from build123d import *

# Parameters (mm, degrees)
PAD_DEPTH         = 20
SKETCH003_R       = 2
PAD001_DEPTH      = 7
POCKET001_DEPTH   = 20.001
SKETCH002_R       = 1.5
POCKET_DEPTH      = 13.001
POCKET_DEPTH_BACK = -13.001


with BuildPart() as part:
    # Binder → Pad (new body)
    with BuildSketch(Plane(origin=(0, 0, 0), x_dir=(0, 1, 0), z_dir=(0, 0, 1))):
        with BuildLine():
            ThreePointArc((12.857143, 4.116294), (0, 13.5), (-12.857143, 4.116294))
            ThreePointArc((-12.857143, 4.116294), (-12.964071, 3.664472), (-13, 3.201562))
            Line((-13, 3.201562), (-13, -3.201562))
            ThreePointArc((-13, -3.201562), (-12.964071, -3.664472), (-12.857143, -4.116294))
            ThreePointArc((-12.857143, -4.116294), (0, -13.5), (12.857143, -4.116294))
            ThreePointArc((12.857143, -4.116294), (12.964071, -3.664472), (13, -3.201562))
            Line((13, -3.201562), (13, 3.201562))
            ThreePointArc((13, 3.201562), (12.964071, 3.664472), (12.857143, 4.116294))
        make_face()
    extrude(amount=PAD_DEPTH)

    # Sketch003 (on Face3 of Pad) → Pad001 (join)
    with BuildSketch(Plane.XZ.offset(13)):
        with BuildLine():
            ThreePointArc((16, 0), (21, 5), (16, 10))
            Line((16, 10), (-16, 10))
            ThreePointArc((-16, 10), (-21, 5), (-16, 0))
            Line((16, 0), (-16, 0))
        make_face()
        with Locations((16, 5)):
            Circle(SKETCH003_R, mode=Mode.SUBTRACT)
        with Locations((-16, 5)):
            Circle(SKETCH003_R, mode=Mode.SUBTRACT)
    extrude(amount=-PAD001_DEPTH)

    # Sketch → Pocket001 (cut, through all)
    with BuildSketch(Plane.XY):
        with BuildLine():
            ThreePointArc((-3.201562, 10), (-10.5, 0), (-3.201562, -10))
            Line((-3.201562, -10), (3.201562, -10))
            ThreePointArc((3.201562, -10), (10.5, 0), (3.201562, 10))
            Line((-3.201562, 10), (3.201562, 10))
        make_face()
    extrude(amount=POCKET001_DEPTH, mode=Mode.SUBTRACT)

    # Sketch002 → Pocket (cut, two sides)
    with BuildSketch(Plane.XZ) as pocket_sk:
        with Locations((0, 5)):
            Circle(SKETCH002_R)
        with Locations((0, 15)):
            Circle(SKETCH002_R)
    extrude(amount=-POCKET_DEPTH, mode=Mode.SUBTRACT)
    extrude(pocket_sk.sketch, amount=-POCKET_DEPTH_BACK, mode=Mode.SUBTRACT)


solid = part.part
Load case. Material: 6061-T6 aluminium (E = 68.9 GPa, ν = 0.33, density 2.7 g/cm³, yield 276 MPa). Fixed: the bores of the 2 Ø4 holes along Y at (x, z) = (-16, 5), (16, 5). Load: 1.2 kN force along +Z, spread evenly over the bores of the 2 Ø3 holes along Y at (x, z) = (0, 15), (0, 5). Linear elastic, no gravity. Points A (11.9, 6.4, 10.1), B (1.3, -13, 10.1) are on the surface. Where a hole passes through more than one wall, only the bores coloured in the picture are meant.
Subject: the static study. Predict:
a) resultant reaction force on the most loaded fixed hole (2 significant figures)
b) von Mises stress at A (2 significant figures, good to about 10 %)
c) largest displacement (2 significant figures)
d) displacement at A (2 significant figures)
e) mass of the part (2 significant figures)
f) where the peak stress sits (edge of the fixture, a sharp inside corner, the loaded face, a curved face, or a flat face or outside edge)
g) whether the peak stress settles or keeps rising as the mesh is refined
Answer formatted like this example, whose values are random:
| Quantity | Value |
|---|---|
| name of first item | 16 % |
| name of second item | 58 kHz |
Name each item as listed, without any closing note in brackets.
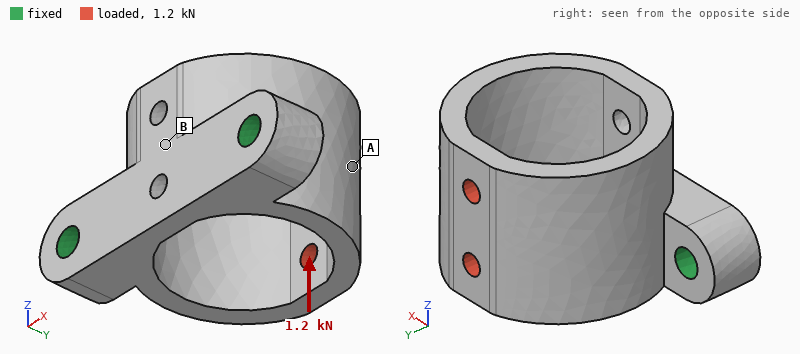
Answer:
| Quantity | Value |
|---|---|
| resultant reaction force on the most loaded fixed hole | 600 N |
| von Mises stress at A | 50 MPa |
| largest displacement | 0.18 mm |
| displacement at A | 0.088 mm |
| mass of the part | 16 g |
| where the peak stress sits | edge of the fixture |
| whether the peak stress settles or keeps rising as the mesh is refined | keeps rising |
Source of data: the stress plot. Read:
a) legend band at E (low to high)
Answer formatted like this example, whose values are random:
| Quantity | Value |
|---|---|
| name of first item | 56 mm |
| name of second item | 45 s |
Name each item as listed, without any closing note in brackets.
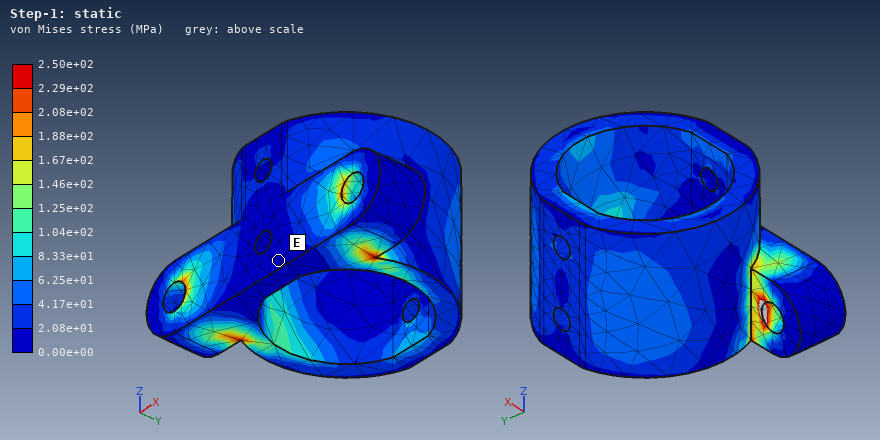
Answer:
| Quantity | Value |
|---|---|
| legend band at E | 0.00e+00 to 2.08e+01 MPa |
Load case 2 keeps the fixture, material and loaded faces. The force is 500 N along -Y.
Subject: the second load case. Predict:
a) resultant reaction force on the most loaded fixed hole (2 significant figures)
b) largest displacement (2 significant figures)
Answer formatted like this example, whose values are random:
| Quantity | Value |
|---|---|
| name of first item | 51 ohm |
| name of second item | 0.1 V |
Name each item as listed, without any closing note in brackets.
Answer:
| Quantity | Value |
|---|---|
| resultant reaction force on the most loaded fixed hole | 270 N |
| largest displacement | 28 µm |
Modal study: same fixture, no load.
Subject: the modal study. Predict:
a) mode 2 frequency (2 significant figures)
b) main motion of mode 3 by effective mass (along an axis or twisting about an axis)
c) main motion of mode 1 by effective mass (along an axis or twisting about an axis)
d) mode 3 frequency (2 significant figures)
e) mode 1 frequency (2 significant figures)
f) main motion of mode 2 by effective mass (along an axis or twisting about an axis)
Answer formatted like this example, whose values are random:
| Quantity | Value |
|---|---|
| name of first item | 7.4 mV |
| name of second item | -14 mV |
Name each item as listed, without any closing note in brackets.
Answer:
| Quantity | Value |
|---|---|
| mode 2 frequency | 7700 Hz |
| main motion of mode 3 by effective mass | twisting about Y |
| main motion of mode 1 by effective mass | along Z |
| mode 3 frequency | 14 kHz |
| mode 1 frequency | 6700 Hz |
| main motion of mode 2 by effective mass | along X |
